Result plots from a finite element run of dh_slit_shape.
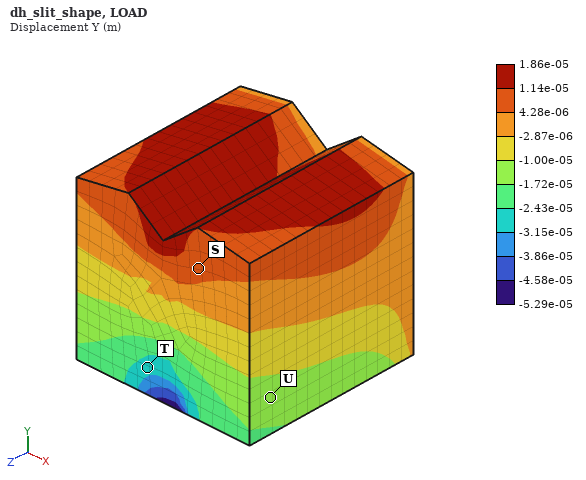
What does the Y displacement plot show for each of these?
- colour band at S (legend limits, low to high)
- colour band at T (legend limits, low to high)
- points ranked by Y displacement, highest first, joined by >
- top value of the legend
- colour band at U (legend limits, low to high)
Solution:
4.28e-06 to 1.14e-05 m
-3.15e-05 to -2.43e-05 m
S > U > T
1.86e-05 m
-1.72e-05 to -1.00e-05 m
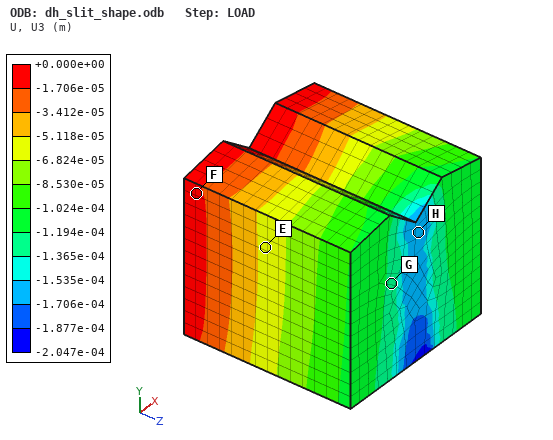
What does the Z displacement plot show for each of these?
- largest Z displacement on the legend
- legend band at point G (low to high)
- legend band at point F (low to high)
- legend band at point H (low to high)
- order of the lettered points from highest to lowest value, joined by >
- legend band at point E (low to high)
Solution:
+0.000e+00 m
-1.365e-04 to -1.194e-04 m
-1.706e-05 to +0.000e+00 m
-1.706e-04 to -1.535e-04 m
F > E > G > H
-6.824e-05 to -5.118e-05 m
